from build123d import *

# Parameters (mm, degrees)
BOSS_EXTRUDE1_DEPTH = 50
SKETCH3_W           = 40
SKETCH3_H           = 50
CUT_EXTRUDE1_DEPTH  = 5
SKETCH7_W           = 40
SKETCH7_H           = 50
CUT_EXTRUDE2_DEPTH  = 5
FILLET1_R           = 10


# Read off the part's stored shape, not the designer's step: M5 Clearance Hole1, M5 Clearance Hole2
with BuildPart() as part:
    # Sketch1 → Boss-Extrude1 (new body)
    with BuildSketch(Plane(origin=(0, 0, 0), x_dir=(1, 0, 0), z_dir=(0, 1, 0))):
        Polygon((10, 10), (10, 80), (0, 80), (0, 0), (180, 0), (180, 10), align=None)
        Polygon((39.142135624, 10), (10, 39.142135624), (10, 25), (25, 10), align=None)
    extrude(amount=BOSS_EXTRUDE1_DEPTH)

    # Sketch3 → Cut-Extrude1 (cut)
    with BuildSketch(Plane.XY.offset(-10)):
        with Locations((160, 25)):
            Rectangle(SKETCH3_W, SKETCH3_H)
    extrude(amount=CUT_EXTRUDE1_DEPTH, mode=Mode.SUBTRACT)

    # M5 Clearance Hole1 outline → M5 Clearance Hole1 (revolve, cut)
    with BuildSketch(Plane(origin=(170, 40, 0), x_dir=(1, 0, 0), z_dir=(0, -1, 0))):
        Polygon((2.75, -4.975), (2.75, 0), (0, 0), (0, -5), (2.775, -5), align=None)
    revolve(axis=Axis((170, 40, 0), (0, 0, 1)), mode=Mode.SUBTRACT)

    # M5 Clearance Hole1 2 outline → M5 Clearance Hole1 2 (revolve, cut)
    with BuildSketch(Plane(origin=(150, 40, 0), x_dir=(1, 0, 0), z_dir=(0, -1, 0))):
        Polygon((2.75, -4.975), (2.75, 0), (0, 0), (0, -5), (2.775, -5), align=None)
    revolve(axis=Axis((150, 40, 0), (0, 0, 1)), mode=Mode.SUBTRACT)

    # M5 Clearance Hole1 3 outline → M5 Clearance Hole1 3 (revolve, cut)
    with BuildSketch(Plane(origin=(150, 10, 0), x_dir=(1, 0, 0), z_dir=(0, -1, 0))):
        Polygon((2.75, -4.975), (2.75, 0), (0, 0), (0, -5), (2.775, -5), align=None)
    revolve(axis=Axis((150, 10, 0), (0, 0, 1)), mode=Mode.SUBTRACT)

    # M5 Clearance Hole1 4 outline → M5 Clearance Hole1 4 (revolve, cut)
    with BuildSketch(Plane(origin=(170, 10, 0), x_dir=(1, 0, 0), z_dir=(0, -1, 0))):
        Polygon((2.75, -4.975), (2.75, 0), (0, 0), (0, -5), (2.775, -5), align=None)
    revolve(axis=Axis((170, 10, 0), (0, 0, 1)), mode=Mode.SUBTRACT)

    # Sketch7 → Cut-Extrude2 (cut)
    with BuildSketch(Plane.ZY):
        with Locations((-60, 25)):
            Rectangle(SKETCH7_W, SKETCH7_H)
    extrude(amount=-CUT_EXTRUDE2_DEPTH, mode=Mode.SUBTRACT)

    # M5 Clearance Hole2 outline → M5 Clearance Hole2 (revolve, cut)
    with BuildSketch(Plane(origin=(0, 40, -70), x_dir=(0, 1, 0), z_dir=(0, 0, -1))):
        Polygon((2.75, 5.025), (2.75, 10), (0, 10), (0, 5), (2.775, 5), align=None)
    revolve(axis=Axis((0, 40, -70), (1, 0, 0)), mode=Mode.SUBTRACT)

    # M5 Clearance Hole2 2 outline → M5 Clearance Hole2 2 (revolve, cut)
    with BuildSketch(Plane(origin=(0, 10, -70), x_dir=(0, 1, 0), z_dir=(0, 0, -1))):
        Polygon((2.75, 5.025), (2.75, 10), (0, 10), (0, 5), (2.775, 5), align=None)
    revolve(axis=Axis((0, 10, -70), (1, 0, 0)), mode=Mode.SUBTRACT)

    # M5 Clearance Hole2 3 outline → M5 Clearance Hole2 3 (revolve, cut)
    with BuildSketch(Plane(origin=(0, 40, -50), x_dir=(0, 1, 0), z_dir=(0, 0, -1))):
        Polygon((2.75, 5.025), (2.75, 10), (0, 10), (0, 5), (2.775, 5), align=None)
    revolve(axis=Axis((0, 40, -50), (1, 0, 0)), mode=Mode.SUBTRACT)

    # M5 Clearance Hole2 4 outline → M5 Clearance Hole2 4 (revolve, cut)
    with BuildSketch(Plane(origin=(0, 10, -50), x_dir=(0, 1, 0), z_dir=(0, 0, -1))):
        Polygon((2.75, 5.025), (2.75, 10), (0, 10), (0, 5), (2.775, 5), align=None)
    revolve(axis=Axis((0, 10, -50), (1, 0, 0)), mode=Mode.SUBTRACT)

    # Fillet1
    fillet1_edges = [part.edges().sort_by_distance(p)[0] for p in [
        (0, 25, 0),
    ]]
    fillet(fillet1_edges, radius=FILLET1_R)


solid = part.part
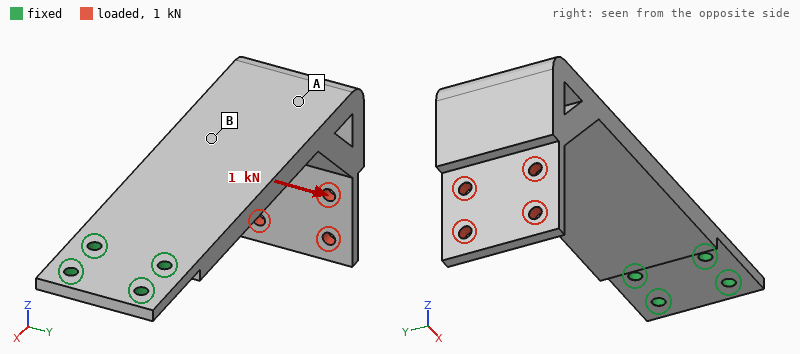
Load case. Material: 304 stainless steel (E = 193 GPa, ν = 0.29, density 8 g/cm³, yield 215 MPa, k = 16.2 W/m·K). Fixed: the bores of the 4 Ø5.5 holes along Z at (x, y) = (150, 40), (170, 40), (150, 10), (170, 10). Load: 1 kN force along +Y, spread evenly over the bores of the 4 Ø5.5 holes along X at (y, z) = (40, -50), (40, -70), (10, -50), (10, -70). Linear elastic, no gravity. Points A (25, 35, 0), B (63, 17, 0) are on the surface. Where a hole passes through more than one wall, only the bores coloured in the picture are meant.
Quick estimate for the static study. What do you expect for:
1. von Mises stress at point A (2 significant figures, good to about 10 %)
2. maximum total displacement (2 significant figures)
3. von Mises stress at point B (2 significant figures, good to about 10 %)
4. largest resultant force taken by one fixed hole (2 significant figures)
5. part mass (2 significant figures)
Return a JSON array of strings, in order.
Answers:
["14 MPa", "0.49 mm", "54 MPa", "4.1 kN", "950 g"]
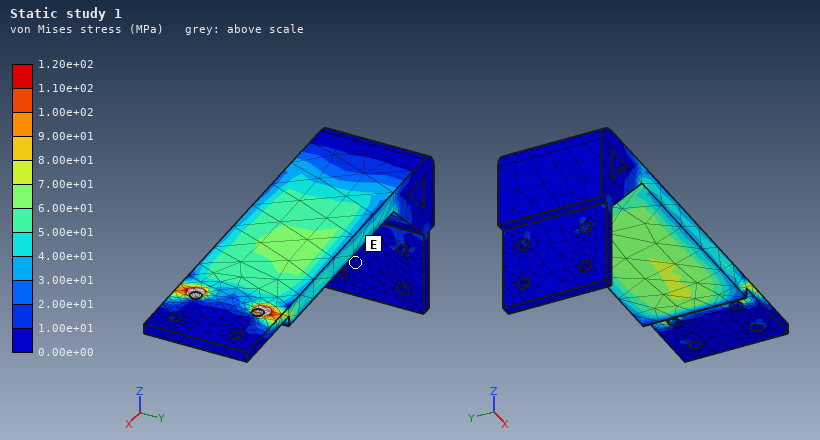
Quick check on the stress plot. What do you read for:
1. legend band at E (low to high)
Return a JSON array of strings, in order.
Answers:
["0.00e+00 to 1.00e+01 MPa"]
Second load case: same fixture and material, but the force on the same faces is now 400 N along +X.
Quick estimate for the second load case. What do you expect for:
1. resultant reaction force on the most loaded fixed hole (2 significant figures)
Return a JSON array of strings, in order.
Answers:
["220 N"]
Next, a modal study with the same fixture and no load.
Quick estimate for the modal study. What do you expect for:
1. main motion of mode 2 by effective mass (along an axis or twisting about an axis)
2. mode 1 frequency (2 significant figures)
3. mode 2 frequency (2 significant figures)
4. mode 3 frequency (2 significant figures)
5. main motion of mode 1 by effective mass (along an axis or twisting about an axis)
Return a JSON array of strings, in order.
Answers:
["along Y", "130 Hz", "650 Hz", "1100 Hz", "along Z"]
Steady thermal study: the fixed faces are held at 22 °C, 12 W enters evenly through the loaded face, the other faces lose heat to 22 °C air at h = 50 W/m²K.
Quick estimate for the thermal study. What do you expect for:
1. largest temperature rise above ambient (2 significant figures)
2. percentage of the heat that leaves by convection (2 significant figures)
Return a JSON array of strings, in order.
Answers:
["44 K", "99 %"]
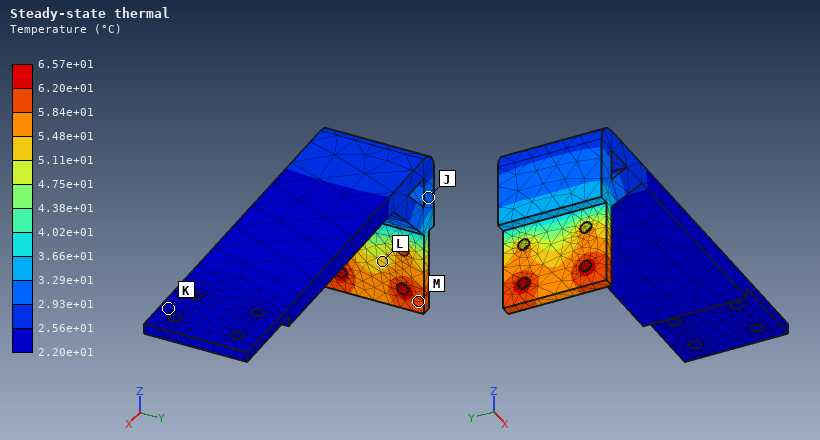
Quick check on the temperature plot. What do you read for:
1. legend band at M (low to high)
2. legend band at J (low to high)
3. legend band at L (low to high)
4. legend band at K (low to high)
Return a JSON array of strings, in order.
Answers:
["5.84e+01 to 6.20e+01 °C", "2.93e+01 to 3.29e+01 °C", "5.11e+01 to 5.48e+01 °C", "2.20e+01 to 2.56e+01 °C"]
